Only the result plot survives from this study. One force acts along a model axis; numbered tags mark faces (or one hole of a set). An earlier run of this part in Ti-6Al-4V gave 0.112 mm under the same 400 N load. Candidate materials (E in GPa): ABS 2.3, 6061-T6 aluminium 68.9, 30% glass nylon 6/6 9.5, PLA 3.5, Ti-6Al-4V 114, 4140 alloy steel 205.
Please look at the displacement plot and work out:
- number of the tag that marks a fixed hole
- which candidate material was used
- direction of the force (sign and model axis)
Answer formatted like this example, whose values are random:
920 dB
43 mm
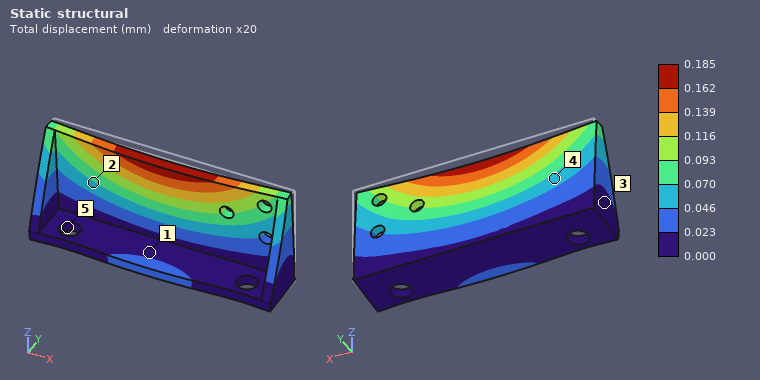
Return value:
5
6061-T6 aluminium
-Y
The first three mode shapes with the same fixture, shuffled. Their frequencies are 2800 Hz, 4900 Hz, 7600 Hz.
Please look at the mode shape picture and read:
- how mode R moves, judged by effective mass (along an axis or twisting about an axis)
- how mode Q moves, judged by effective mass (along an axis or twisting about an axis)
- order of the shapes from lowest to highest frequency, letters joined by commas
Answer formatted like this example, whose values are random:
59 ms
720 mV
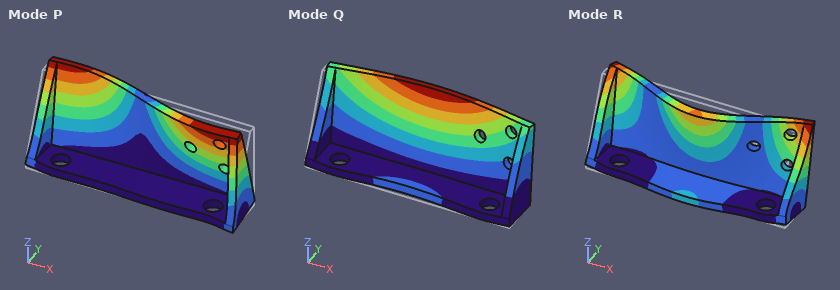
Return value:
along Z
along Y
Q, P, R
